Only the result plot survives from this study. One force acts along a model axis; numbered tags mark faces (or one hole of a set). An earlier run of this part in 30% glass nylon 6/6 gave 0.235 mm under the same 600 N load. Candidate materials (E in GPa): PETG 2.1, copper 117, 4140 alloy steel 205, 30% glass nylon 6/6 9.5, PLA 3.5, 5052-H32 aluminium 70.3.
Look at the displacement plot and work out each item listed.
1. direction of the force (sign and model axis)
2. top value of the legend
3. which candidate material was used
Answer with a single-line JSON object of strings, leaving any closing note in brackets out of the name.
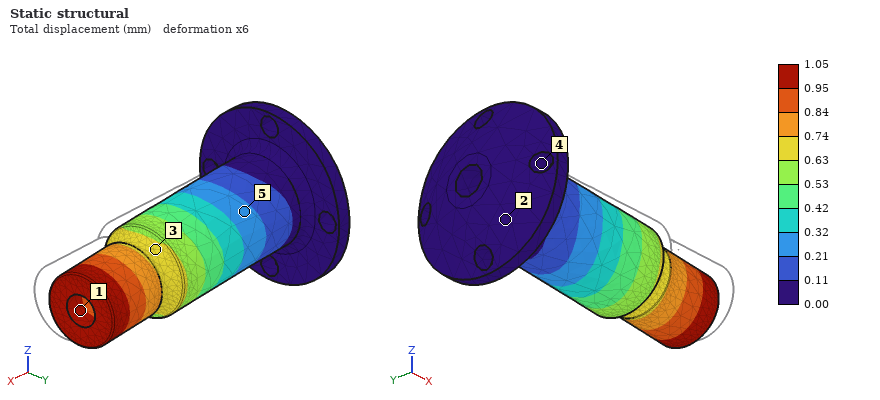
{"direction of the force": "+Y", "top value of the legend": "1.05 mm", "which candidate material was used": "PETG"}
